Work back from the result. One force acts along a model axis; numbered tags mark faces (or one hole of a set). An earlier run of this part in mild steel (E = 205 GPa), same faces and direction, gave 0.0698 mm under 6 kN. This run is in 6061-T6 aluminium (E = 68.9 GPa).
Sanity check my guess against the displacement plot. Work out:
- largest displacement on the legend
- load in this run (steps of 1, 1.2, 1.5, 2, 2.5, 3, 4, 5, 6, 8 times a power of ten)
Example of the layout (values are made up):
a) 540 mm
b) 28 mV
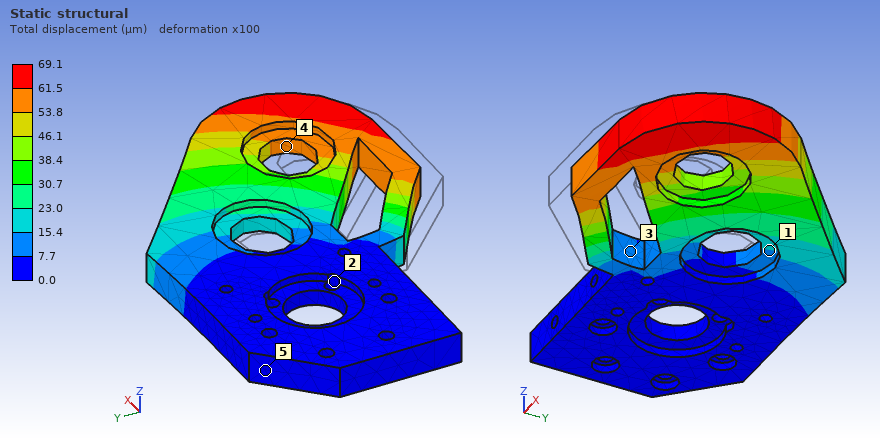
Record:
a) 69.1 µm
b) 2 kN
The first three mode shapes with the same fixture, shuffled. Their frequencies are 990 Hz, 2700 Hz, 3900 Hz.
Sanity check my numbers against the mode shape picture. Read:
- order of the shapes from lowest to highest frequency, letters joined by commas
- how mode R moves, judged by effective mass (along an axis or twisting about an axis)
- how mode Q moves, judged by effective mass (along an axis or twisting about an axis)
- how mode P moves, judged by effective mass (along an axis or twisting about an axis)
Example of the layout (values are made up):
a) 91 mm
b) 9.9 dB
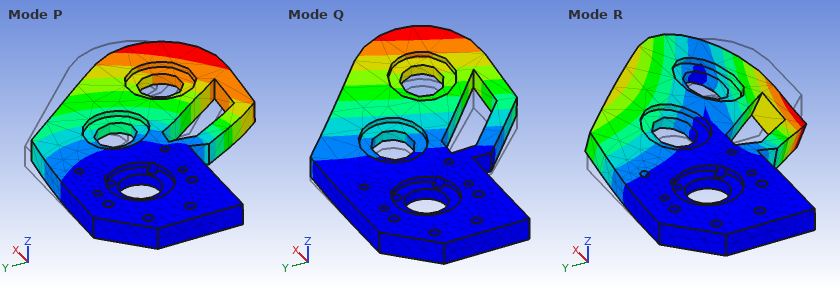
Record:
a) Q, R, P
b) twisting about X
c) along Z
d) along Y
